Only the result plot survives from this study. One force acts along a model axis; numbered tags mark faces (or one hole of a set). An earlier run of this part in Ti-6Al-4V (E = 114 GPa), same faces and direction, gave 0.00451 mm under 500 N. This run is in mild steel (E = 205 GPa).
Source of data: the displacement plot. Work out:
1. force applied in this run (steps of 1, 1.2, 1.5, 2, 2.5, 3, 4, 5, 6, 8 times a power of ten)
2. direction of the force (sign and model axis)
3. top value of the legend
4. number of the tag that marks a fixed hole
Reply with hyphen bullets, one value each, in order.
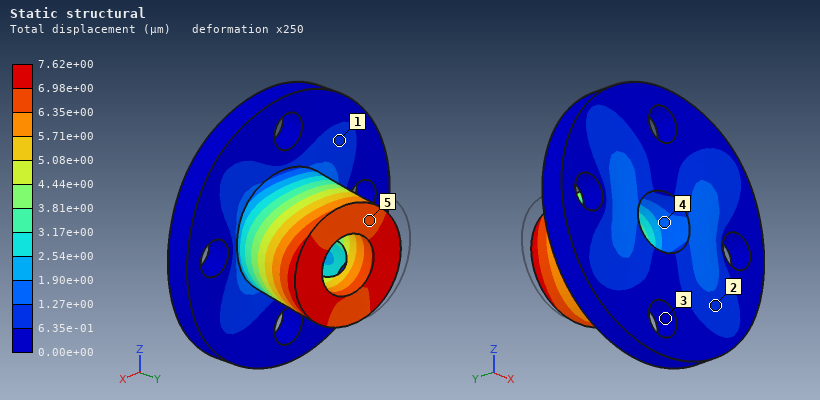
- 1.5 kN
- +X
- 7.62e+00 µm
- 3
